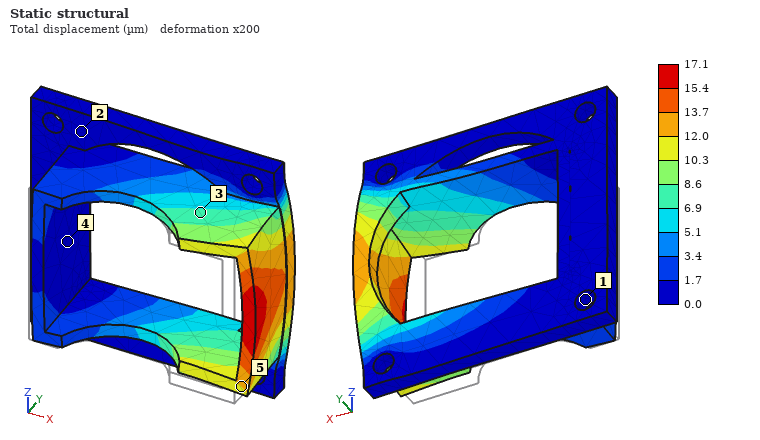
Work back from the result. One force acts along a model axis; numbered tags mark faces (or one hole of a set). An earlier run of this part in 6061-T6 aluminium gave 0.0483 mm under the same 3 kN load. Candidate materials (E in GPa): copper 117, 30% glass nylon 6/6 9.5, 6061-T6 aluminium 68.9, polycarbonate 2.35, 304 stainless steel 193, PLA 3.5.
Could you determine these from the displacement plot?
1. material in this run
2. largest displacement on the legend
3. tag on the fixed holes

304 stainless steel
17.1 µm
1
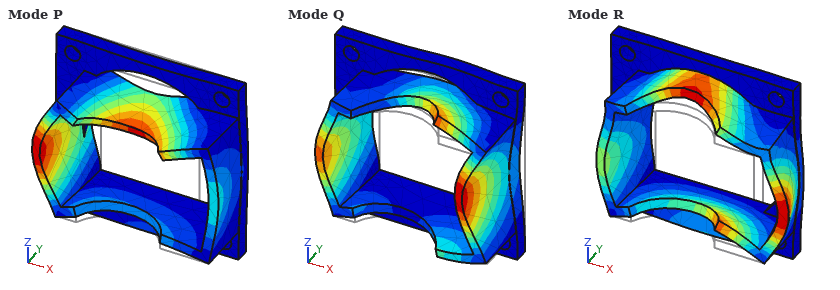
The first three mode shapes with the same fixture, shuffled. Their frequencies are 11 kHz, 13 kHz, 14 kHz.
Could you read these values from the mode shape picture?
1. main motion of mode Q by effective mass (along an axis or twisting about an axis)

along X
